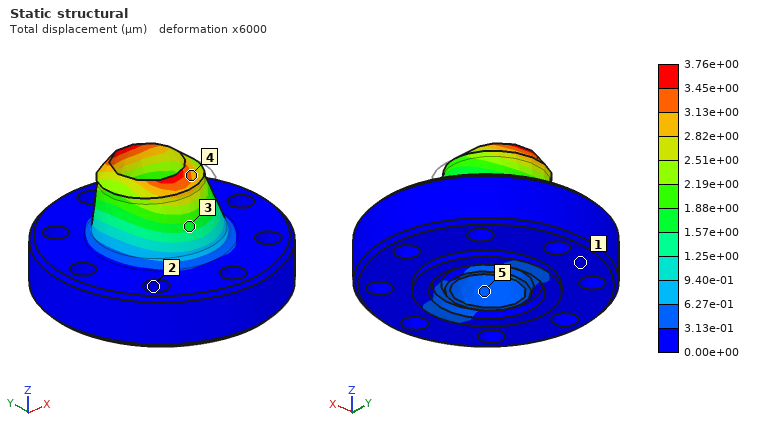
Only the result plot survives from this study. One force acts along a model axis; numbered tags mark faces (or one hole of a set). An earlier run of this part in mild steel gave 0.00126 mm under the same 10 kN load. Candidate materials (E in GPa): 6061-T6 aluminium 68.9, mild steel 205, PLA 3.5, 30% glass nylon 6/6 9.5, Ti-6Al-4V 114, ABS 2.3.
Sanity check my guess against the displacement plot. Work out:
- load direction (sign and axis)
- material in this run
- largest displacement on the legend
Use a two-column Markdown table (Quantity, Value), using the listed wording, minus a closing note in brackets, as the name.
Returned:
| Quantity | Value |
|---|---|
| load direction | +Y |
| material in this run | 6061-T6 aluminium |
| largest displacement on the legend | 3.76e+00 µm |
